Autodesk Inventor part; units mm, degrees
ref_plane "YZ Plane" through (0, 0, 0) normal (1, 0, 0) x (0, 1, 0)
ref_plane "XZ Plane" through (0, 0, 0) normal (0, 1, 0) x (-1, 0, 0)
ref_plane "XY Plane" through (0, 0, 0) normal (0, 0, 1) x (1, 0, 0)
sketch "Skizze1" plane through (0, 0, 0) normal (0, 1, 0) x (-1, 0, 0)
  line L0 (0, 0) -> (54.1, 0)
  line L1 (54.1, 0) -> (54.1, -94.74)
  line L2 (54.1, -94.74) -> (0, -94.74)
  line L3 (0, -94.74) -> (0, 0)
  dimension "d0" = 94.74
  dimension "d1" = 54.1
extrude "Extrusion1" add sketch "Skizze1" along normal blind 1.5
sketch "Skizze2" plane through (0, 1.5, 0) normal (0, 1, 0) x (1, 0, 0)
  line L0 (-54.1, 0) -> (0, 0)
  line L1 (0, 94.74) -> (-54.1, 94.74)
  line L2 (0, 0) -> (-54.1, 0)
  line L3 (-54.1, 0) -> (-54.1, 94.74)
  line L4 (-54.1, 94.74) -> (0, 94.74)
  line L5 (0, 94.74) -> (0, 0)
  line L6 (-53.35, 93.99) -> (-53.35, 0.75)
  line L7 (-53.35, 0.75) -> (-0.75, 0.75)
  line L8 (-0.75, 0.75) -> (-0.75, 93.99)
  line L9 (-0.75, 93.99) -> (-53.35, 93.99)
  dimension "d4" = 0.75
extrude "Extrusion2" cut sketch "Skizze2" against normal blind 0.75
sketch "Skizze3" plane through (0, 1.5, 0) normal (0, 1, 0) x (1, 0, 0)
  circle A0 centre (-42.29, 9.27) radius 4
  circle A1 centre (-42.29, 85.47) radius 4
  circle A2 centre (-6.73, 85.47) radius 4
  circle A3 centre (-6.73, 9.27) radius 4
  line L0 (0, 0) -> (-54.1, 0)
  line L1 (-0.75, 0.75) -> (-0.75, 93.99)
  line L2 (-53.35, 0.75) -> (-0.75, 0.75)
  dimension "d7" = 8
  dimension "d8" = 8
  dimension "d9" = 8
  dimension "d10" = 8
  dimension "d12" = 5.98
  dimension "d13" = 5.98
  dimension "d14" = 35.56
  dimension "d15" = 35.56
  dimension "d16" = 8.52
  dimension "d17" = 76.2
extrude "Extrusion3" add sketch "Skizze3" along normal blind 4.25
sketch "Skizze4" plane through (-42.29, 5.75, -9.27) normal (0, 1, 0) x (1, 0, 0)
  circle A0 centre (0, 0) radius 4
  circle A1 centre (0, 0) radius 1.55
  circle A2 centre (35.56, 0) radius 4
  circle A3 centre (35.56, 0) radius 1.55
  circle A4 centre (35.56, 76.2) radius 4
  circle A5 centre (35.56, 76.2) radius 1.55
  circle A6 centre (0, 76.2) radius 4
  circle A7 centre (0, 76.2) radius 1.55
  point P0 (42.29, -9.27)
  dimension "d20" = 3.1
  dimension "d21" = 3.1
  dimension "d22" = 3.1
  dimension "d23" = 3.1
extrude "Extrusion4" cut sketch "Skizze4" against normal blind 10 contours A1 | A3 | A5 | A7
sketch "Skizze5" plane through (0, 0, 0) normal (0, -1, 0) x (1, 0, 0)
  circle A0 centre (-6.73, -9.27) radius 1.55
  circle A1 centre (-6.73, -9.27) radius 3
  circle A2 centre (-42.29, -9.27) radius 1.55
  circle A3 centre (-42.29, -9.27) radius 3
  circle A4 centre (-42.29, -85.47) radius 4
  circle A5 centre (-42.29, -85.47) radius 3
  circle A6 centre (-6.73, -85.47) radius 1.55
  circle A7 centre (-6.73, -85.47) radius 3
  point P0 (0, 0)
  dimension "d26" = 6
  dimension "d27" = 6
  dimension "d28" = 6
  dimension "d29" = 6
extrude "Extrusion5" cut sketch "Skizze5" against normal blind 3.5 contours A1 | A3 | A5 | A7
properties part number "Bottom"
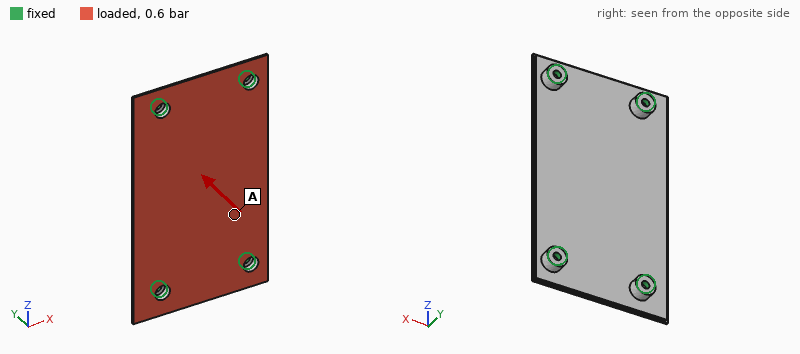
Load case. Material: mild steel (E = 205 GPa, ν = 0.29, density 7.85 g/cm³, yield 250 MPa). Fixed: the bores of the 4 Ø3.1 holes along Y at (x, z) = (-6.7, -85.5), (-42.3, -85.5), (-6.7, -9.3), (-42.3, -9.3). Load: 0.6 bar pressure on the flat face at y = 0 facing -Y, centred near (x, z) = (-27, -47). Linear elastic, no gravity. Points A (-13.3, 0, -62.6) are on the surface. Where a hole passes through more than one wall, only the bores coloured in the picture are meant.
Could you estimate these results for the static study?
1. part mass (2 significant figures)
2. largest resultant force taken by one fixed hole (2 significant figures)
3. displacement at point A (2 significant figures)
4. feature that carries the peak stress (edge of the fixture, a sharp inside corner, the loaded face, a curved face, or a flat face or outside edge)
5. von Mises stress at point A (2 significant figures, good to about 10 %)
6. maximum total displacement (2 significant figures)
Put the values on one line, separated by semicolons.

62 g; 140 N; 62 µm; a curved face; 21 MPa; 94 µm
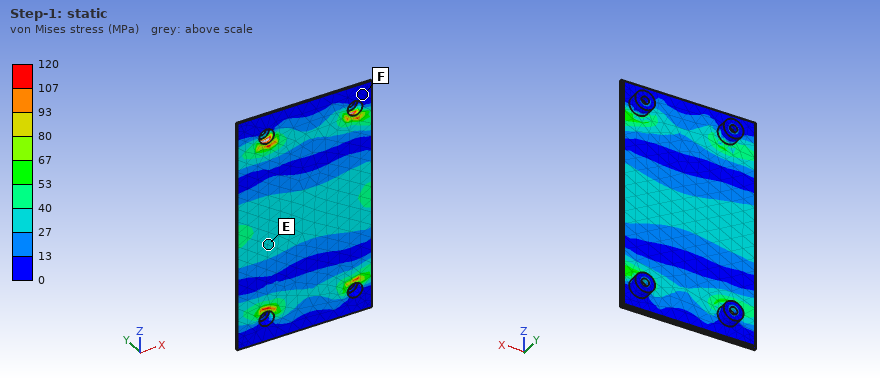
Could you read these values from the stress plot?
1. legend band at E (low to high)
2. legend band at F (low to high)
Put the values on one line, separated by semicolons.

27 to 40 MPa; 0 to 13 MPa
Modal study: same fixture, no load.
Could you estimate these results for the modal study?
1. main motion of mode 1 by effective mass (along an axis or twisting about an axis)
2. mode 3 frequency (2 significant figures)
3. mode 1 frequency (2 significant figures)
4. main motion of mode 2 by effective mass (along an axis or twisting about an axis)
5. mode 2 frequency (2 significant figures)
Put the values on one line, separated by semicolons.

along Y; 3700 Hz; 1400 Hz; twisting about Z; 2000 Hz
